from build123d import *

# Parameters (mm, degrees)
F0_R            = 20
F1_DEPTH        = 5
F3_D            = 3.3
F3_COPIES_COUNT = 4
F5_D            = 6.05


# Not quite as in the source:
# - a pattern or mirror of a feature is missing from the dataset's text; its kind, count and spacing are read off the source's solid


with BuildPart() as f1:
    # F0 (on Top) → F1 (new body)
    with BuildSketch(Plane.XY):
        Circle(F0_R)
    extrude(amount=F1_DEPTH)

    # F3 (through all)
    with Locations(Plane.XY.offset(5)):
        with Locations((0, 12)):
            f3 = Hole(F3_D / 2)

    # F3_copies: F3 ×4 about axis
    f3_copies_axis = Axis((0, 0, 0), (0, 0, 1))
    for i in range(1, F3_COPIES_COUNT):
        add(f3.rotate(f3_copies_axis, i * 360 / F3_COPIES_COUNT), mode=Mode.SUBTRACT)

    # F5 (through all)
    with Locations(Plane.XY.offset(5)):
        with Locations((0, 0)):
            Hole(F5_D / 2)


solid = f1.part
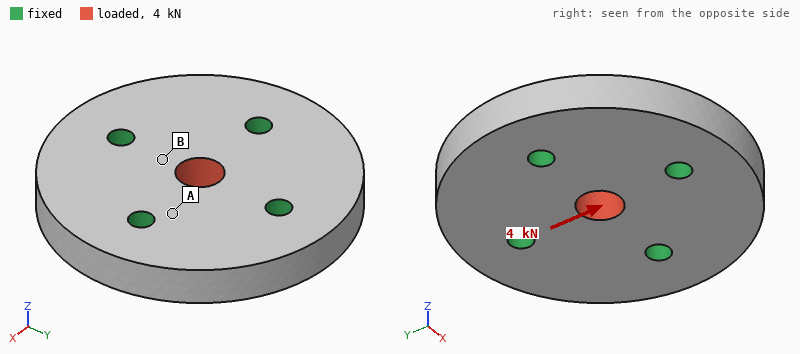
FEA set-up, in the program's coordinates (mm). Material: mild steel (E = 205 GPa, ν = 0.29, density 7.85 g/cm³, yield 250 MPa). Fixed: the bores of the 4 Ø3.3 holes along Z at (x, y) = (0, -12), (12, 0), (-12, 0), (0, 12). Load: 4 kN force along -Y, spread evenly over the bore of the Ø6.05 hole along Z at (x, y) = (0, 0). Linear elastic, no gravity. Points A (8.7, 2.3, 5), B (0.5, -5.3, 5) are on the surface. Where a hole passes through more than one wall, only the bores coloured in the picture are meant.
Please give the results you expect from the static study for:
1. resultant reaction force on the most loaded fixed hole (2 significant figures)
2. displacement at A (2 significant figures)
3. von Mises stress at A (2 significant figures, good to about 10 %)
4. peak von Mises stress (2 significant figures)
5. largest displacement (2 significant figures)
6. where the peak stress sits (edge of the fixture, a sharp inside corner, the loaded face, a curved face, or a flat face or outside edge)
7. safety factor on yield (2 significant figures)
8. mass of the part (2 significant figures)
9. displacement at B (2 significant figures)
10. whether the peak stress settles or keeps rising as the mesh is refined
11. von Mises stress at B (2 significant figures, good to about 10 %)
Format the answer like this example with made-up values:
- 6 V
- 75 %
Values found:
- 1.3 kN
- 0.38 µm
- 11 MPa
- 73 MPa
- 1.7 µm
- the loaded face
- 3.4
- 47 g
- 1.1 µm
- settles
- 43 MPa
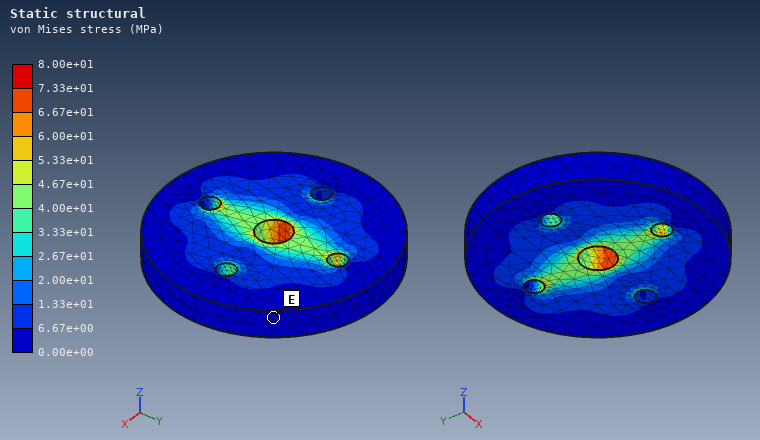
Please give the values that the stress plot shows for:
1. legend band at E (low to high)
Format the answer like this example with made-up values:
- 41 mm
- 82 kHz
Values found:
- 0.00e+00 to 6.67e+00 MPa
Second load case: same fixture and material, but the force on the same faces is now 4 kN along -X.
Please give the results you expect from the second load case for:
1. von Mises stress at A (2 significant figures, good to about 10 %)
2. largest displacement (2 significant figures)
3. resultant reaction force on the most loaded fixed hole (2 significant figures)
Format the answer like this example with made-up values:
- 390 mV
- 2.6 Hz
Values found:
- 27 MPa
- 1.7 µm
- 1.3 kN
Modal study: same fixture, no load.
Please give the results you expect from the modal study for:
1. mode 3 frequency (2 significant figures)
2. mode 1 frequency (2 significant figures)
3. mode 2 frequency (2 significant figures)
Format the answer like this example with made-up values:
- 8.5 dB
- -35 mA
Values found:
- 32 kHz
- 30 kHz
- 32 kHz
